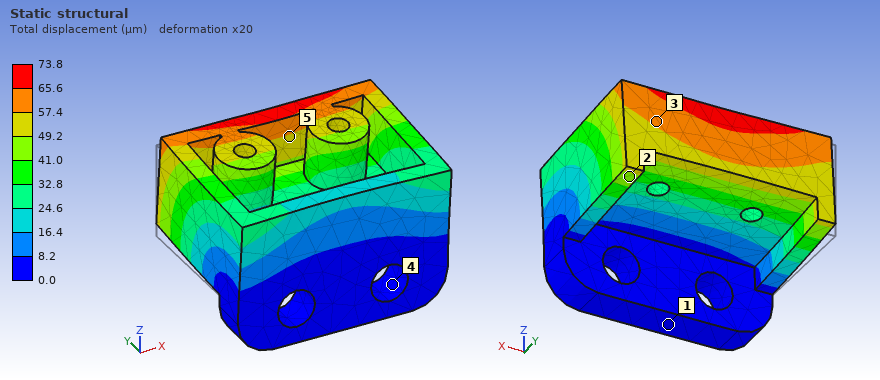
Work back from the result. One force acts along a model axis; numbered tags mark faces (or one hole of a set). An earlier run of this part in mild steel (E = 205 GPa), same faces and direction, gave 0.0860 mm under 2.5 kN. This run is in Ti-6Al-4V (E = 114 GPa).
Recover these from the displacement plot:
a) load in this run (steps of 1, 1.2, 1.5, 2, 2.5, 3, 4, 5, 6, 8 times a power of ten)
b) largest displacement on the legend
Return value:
1.2 kN
73.8 µm
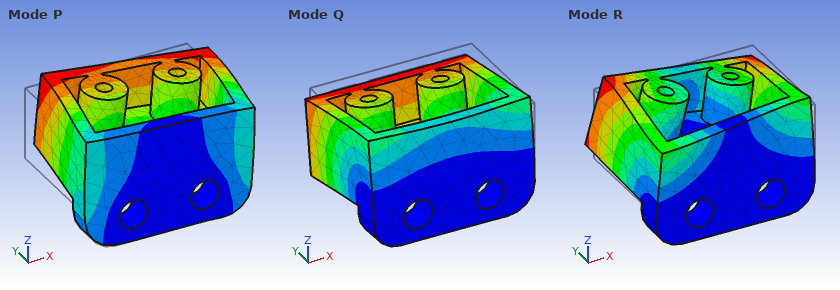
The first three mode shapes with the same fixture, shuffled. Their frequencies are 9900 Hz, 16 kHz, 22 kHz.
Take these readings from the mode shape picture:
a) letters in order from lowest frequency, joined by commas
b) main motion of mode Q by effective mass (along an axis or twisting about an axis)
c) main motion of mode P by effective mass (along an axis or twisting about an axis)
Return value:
Q, R, P
along Z
along X
